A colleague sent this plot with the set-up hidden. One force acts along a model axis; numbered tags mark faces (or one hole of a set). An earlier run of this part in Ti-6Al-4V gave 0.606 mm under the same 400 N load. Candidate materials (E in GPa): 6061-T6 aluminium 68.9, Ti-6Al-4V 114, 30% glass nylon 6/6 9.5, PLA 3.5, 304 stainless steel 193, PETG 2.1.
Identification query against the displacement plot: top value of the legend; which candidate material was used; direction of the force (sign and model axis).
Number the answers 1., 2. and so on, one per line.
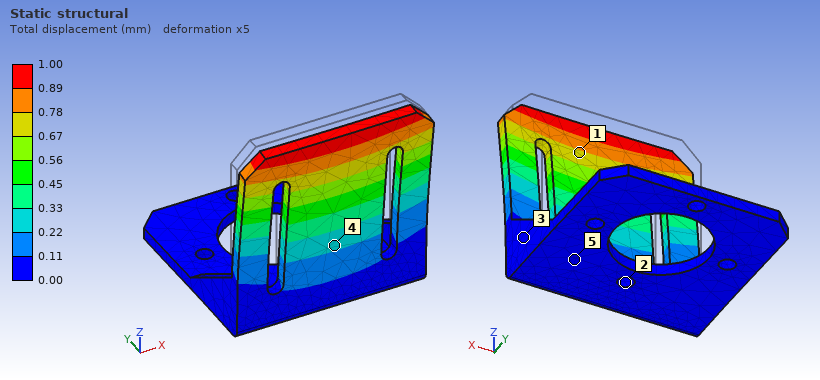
1. 1.00 mm
2. 6061-T6 aluminium
3. -Y
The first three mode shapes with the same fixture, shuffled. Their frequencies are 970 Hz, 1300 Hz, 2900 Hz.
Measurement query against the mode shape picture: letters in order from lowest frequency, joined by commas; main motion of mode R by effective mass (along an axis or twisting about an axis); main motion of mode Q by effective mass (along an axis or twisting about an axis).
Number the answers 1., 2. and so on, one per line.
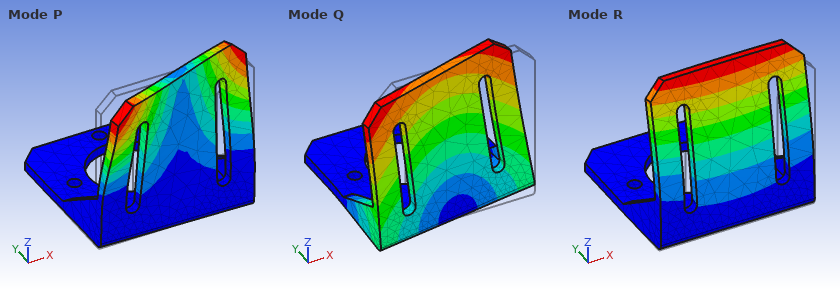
1. R, Q, P
2. along Y
3. along X
